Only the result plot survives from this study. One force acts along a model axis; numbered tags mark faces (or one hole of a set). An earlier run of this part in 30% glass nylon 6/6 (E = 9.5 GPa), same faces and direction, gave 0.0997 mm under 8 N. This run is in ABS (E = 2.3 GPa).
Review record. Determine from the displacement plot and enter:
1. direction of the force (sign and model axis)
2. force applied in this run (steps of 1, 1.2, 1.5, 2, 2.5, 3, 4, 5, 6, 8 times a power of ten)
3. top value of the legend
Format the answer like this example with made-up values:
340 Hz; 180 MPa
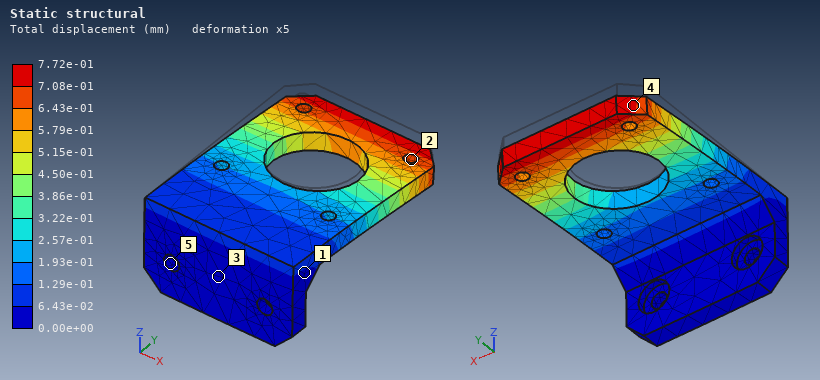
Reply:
-Z; 15 N; 7.72e-01 mm
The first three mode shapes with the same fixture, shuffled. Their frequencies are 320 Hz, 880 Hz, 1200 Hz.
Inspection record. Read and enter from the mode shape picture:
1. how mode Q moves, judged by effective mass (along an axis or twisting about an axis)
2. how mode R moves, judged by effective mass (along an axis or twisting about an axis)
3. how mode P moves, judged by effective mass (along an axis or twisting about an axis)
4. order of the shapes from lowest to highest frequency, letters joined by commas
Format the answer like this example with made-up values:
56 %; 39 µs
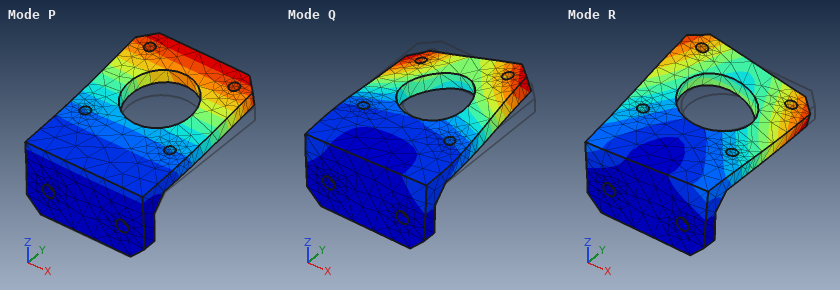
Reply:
along X; along X; along Z; P, R, Q
